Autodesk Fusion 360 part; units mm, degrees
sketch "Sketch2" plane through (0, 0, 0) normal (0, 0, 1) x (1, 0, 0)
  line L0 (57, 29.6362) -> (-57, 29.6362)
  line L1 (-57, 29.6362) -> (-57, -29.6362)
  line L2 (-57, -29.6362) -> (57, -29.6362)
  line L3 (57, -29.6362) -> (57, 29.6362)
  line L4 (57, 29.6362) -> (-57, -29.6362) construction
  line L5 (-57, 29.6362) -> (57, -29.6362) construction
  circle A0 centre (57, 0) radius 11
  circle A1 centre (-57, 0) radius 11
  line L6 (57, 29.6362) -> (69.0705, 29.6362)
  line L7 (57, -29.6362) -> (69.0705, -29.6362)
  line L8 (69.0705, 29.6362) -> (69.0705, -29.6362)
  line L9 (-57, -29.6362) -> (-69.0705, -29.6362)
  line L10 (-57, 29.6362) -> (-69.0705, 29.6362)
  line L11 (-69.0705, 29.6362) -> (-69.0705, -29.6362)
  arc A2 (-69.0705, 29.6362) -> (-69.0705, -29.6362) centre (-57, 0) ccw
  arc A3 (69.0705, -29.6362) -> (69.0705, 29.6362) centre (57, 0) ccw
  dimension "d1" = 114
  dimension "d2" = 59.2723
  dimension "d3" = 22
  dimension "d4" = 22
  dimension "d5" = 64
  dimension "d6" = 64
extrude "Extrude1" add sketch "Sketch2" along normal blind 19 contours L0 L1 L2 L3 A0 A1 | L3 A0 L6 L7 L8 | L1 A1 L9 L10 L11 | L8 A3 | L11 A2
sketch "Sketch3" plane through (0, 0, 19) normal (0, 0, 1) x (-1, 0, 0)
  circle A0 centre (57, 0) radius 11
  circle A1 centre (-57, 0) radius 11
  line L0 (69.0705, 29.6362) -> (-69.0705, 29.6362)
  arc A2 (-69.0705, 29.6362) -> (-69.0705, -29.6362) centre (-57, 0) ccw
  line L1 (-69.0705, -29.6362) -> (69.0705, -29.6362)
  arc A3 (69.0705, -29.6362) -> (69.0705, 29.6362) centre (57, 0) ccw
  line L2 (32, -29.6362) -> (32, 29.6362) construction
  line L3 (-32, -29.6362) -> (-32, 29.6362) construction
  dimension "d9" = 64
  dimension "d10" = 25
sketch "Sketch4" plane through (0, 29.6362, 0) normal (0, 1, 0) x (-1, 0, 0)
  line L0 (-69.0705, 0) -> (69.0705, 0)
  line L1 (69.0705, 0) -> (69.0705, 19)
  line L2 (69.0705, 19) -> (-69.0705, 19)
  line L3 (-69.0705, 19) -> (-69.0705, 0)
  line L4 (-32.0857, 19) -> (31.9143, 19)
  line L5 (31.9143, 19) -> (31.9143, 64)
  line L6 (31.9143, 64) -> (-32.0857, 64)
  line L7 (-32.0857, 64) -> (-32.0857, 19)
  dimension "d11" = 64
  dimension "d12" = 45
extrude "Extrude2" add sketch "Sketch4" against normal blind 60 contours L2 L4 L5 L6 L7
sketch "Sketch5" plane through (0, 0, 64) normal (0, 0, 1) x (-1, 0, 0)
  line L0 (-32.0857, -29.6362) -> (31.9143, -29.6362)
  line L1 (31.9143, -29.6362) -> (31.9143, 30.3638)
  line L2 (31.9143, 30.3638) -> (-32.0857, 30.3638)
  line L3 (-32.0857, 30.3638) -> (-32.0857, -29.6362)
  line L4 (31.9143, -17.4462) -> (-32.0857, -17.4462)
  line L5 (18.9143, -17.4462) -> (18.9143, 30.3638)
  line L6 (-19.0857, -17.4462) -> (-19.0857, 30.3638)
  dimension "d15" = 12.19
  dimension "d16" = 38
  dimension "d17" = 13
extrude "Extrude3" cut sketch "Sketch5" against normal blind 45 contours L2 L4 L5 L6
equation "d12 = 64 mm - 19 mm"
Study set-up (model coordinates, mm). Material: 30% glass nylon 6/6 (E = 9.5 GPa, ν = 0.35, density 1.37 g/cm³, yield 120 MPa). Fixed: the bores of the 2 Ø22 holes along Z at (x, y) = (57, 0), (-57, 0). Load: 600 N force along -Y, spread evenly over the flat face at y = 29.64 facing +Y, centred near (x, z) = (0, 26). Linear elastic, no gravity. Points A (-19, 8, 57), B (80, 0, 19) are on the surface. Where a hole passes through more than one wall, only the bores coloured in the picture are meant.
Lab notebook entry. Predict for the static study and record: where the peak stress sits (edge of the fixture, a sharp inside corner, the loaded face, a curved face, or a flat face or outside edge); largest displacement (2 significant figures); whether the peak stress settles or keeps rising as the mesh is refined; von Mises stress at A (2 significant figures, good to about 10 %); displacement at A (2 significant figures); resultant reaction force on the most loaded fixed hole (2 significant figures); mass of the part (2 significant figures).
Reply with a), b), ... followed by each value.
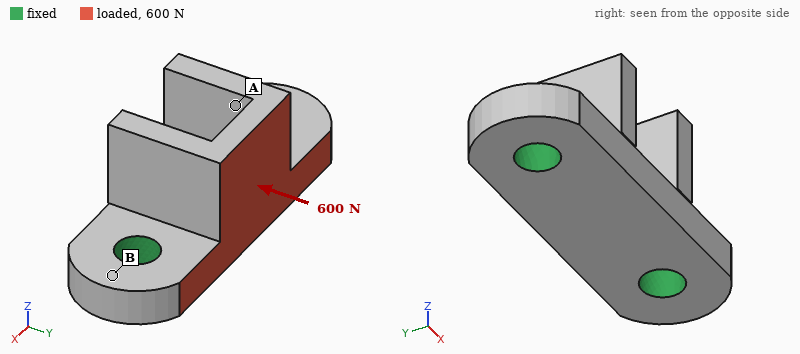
a) edge of the fixture
b) 22 µm
c) keeps rising
d) 0.48 MPa
e) 16 µm
f) 300 N
g) 360 g
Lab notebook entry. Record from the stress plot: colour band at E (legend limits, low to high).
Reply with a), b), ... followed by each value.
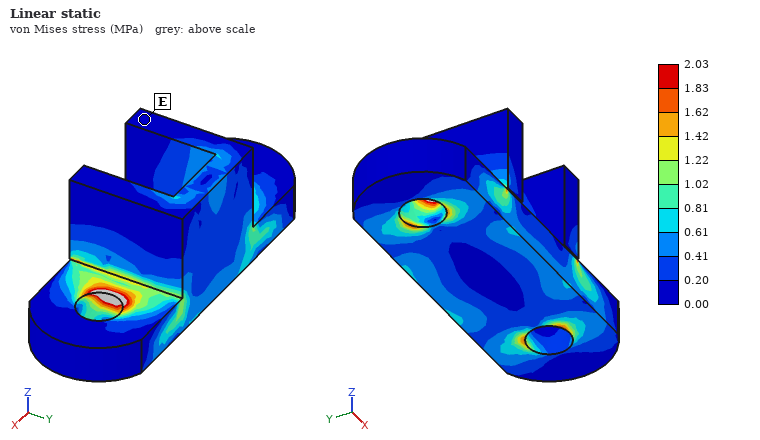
a) 0.00 to 0.20 MPa
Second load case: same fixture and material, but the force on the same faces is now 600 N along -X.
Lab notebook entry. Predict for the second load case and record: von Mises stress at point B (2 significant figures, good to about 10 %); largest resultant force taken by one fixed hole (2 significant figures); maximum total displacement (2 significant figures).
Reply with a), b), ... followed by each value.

a) 0.084 MPa
b) 350 N
c) 8.4 µm
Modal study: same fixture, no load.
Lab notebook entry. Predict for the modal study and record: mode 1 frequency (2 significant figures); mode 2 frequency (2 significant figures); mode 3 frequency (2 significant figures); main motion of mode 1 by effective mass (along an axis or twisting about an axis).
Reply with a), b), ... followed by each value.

a) 2000 Hz
b) 2800 Hz
c) 2900 Hz
d) along Y
